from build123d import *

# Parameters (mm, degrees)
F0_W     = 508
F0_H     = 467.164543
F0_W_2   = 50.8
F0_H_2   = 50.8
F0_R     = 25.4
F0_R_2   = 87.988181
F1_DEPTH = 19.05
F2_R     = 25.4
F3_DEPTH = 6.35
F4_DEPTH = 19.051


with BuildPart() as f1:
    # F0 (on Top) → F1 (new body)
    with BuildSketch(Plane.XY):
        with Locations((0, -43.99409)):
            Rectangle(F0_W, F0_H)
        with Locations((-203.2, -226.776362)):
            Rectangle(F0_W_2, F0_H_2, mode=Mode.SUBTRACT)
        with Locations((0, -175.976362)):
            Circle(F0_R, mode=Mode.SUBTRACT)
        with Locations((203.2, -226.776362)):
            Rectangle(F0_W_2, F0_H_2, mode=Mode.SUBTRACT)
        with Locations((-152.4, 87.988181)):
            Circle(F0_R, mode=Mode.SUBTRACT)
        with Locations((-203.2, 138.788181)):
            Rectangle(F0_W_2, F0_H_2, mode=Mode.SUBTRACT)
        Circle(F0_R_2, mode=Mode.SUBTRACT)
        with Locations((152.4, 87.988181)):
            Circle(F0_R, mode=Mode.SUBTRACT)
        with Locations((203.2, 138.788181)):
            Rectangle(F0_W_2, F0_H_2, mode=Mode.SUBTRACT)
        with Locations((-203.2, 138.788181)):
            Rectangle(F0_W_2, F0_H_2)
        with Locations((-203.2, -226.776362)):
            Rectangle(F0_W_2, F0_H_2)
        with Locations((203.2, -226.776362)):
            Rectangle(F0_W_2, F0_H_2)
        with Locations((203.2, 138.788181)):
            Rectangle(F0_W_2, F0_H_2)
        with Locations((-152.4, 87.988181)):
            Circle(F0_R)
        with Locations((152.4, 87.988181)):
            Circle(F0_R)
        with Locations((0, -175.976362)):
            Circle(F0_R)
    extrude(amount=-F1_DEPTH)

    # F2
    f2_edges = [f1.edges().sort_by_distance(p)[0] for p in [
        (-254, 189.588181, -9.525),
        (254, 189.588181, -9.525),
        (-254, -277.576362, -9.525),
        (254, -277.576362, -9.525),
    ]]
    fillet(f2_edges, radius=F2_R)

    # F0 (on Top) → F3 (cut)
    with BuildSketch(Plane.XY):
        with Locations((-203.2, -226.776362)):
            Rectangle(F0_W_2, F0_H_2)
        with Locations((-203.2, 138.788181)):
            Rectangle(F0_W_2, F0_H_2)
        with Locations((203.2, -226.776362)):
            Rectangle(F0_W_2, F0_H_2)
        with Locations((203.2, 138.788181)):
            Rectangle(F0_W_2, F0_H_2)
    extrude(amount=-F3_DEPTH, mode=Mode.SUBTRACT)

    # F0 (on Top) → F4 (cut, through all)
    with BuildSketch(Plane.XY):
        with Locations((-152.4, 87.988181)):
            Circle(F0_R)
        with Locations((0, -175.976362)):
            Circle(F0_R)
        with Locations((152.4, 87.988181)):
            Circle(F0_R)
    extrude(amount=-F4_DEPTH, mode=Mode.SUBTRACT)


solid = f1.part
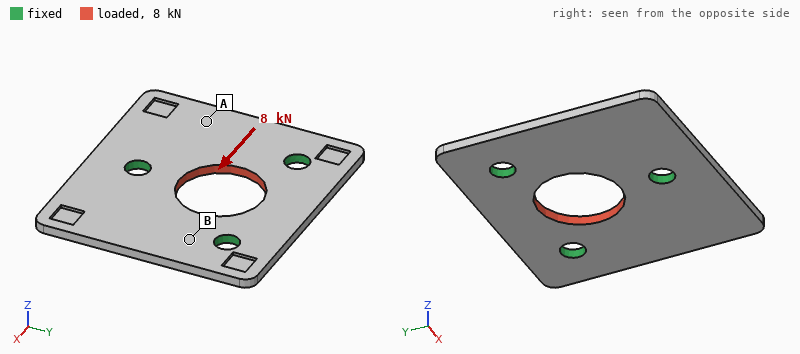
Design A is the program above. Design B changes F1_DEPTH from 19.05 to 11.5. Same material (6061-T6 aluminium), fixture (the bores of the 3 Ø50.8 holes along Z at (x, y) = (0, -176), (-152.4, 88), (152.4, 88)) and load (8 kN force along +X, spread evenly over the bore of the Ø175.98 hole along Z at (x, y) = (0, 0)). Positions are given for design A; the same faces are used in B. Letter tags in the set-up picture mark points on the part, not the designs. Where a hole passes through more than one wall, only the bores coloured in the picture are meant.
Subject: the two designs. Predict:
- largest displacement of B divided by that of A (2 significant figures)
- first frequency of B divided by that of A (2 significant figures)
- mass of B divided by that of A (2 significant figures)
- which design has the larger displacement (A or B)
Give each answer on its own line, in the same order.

1.7
0.63
0.60
B
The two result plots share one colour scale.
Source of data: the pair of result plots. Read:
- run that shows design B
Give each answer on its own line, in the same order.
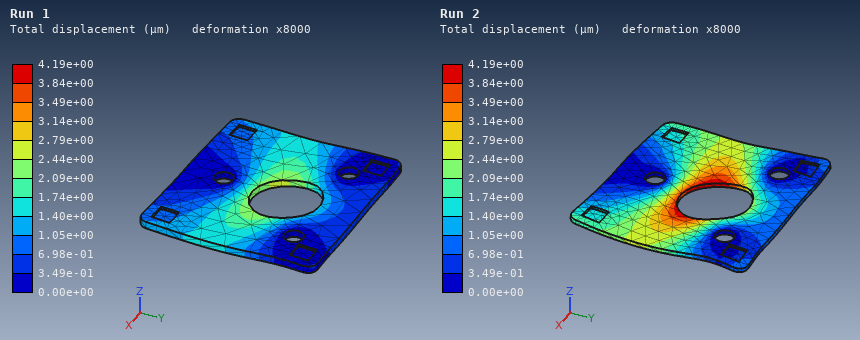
Run 2
